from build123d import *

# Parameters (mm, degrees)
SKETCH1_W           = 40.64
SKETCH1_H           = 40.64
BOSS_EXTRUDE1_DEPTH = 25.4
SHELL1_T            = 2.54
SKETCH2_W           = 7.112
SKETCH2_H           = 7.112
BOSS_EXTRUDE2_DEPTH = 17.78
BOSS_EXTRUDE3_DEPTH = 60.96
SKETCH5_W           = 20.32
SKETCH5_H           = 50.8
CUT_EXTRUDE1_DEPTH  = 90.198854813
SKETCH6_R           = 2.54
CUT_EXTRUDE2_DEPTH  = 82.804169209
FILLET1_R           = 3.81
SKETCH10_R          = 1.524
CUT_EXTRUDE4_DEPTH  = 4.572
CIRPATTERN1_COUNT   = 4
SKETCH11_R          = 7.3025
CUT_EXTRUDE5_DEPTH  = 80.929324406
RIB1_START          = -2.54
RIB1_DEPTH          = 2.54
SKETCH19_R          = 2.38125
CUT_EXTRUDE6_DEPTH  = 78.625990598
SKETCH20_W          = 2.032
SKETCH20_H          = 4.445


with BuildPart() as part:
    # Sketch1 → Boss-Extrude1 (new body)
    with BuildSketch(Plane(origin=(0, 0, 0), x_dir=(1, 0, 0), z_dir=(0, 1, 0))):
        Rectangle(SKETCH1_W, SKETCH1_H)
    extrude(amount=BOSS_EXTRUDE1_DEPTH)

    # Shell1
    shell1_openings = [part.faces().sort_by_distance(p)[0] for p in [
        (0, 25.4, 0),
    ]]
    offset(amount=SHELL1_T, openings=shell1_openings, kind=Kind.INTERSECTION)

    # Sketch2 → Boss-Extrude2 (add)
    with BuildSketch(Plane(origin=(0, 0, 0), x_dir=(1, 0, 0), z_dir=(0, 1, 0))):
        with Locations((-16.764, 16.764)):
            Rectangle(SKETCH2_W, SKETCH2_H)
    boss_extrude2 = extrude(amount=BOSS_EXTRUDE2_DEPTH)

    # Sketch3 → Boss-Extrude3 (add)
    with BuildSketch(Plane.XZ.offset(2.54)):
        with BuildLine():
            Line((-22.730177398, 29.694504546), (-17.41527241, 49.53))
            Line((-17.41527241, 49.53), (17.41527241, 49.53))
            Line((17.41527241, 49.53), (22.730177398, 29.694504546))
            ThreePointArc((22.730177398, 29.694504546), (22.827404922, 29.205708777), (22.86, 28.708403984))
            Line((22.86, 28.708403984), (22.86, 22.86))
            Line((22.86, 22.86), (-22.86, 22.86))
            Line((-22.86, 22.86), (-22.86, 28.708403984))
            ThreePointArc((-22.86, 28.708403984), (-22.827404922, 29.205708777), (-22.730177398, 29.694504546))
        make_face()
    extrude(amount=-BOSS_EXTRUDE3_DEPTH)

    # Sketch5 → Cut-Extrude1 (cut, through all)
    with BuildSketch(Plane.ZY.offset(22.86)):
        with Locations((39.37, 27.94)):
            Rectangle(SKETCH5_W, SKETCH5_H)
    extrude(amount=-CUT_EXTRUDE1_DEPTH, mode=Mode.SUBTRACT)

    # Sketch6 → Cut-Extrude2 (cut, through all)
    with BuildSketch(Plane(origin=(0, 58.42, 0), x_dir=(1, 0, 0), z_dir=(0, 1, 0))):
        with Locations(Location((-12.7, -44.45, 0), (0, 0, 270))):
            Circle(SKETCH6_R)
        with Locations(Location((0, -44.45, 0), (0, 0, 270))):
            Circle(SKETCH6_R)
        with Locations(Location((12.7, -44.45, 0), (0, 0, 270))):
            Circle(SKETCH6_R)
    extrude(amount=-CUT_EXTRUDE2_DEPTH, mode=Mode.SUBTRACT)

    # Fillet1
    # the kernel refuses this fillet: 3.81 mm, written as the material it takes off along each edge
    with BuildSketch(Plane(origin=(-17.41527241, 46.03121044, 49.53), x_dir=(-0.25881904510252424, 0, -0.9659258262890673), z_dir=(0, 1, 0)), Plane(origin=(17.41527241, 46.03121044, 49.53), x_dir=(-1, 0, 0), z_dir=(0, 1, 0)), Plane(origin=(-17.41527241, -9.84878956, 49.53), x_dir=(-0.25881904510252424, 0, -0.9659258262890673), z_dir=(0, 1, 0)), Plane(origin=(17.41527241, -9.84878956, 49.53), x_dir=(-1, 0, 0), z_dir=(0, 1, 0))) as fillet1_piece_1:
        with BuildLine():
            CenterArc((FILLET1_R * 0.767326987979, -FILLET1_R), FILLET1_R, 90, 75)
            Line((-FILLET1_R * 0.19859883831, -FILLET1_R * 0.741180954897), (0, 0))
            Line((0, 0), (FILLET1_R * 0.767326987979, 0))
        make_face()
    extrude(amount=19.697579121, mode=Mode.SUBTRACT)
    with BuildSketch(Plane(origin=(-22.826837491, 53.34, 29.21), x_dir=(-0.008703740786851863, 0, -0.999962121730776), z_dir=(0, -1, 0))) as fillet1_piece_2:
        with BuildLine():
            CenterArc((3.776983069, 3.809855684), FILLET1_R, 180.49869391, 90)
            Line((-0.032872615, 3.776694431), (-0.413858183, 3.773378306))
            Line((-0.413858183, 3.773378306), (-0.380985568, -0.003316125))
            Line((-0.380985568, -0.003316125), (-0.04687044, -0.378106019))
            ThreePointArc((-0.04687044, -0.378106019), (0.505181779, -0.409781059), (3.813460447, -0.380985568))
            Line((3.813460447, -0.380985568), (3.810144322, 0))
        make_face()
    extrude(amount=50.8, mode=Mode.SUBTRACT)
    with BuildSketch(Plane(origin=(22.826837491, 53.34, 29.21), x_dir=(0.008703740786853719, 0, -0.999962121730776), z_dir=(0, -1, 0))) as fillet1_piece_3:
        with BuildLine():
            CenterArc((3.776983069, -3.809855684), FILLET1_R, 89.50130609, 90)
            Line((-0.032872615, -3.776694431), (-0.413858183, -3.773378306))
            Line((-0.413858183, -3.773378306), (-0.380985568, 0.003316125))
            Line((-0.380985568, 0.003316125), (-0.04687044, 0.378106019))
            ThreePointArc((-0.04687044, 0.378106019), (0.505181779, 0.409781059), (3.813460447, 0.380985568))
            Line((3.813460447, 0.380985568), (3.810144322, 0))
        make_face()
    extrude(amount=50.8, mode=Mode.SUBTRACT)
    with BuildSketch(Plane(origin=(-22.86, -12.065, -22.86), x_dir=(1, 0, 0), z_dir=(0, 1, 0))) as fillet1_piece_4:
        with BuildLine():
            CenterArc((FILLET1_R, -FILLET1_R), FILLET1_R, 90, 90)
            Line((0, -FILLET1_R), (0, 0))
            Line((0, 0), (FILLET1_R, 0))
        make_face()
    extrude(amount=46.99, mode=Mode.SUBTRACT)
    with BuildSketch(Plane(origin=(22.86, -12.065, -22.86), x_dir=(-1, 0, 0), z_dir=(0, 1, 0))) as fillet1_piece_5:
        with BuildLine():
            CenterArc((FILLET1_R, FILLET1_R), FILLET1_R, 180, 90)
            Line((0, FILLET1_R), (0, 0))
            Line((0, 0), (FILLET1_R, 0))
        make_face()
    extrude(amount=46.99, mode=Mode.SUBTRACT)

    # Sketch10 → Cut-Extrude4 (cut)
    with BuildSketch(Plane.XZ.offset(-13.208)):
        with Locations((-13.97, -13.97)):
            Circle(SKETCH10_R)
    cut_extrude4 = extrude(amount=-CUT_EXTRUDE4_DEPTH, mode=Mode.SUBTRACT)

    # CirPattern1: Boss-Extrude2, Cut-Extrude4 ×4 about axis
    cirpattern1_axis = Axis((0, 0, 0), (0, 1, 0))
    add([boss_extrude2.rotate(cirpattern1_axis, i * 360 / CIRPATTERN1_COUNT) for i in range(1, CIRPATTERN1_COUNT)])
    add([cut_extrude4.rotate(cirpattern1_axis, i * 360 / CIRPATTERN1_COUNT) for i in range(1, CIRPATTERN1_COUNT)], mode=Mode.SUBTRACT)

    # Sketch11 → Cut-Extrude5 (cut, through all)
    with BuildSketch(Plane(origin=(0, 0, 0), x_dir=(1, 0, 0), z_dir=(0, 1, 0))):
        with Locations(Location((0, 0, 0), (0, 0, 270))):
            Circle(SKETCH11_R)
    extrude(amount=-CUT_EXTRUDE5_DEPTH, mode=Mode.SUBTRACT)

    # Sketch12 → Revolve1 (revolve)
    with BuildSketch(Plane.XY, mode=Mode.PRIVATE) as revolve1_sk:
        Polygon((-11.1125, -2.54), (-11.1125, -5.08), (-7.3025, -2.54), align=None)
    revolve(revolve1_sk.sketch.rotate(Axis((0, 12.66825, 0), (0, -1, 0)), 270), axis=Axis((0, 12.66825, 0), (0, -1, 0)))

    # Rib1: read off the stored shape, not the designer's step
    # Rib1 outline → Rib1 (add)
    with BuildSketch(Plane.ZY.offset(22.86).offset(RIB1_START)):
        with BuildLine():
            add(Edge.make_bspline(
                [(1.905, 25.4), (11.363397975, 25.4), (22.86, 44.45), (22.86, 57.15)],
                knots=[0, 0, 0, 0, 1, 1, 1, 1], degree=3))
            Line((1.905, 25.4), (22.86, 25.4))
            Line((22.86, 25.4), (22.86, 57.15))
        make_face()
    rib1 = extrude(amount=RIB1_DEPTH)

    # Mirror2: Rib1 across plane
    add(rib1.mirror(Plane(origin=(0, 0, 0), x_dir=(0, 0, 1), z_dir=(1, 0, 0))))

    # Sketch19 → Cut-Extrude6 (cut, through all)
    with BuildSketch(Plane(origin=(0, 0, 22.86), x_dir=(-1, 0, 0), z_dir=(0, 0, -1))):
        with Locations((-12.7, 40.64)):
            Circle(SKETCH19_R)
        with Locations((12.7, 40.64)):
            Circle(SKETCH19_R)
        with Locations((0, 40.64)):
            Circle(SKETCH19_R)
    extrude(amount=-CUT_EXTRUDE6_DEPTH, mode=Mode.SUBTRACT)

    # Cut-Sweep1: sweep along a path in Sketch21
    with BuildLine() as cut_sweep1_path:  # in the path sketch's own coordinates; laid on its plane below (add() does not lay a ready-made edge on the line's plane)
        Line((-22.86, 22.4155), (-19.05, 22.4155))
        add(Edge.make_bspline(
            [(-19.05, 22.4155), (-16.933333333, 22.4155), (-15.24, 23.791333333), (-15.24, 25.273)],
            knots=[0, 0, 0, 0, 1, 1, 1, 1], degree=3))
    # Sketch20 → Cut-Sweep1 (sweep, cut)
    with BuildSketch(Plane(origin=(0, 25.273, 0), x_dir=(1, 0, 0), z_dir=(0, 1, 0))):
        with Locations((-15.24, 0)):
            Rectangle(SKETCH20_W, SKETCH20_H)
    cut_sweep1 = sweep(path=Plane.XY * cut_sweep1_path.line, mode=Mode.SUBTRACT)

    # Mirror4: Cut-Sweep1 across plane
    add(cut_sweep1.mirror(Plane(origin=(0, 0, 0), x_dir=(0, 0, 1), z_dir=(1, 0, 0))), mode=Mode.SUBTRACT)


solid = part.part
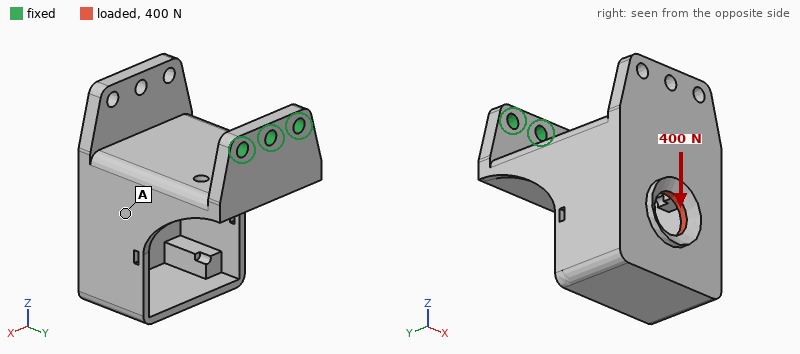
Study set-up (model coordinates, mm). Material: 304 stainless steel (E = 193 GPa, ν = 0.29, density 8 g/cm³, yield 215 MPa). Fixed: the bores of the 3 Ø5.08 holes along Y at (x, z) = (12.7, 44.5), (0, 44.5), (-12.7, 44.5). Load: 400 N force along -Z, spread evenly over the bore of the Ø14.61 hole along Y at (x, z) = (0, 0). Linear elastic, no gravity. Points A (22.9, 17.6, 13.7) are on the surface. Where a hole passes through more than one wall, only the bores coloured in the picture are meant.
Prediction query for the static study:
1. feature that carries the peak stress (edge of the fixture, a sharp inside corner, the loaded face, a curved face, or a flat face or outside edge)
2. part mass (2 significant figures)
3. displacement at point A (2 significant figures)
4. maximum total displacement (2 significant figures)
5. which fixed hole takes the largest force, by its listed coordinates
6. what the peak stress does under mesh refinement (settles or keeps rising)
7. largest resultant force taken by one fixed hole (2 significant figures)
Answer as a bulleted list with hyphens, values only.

- edge of the fixture
- 360 g
- 0.23 mm
- 0.46 mm
- (0, 44.5)
- keeps rising
- 190 N
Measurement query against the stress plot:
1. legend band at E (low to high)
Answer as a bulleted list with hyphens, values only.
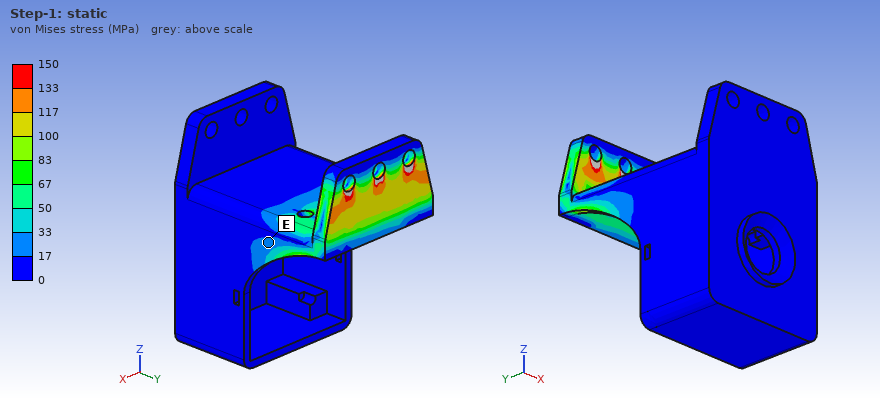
- 17 to 33 MPa
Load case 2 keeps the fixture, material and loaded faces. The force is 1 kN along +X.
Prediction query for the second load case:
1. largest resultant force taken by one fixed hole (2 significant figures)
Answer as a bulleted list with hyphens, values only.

- 2.4 kN
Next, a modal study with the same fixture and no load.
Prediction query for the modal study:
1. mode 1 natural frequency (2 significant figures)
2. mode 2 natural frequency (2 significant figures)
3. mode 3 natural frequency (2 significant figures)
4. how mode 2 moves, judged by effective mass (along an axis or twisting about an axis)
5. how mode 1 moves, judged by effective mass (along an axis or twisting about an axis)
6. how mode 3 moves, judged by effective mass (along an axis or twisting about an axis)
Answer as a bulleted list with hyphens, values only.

- 350 Hz
- 930 Hz
- 1200 Hz
- along X
- along Z
- twisting about Y
